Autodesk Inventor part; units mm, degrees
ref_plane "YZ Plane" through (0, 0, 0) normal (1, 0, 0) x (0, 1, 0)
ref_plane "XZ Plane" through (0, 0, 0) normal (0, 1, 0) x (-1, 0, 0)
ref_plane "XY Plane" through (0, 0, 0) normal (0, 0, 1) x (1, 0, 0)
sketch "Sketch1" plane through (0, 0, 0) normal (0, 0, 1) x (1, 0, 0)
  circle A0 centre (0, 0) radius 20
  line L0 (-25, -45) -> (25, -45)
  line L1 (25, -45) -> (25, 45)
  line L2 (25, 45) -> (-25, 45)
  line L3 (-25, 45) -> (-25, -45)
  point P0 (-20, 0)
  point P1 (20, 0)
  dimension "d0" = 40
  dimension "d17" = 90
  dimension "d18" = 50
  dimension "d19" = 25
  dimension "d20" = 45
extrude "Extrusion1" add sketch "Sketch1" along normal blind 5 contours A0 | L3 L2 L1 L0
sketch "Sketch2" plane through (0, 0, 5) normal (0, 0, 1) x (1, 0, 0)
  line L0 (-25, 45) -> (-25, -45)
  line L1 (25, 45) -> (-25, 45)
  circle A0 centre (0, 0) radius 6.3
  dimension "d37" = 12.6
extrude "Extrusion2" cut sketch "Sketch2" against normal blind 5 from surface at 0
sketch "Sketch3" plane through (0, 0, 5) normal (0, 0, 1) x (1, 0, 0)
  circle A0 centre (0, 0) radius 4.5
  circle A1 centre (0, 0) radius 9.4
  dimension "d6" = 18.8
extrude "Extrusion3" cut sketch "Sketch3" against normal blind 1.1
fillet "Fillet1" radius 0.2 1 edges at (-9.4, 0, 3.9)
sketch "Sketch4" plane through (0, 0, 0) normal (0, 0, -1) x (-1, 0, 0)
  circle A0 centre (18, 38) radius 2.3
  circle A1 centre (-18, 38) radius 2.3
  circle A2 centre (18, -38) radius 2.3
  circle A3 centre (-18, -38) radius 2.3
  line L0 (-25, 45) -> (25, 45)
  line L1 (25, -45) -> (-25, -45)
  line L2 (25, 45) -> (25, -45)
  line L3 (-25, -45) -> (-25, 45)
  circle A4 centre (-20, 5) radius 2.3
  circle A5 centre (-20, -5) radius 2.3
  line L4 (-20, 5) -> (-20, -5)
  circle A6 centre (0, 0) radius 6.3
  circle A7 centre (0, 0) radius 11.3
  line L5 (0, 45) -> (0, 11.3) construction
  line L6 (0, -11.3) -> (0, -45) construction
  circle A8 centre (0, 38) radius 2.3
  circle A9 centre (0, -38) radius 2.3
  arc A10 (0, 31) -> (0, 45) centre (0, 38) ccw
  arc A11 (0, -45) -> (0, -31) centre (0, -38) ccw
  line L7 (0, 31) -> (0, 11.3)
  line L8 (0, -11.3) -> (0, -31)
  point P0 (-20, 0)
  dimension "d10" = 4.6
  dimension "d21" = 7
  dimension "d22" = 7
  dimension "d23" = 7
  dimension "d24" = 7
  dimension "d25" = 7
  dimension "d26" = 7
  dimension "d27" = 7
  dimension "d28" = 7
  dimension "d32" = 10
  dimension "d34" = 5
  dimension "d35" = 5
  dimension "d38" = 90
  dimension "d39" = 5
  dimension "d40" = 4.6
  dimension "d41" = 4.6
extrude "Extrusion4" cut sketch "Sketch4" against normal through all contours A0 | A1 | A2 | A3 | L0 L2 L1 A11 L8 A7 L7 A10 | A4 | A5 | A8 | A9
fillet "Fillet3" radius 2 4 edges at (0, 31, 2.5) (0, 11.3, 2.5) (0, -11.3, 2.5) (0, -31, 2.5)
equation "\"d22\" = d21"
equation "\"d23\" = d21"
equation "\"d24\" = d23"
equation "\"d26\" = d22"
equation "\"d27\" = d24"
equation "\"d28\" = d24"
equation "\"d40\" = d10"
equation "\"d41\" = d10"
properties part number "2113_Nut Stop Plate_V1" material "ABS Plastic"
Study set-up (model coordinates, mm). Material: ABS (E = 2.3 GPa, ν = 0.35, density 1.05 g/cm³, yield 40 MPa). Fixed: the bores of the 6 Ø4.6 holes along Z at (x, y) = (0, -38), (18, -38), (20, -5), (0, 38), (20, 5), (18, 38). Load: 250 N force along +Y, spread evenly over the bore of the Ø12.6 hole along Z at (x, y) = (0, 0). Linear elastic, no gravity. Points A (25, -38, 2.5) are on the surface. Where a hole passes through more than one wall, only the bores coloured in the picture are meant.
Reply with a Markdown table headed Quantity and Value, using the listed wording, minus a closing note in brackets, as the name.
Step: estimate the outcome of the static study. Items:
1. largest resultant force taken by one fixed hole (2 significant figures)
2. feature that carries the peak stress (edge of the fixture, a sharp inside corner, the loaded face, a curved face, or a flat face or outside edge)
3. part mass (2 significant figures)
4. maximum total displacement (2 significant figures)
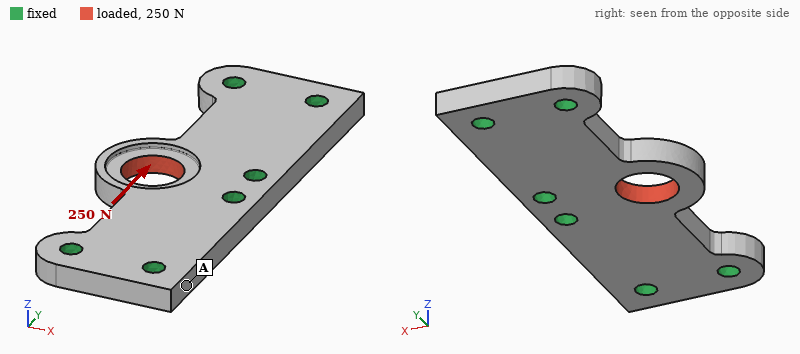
| Quantity | Value |
|---|---|
| largest resultant force taken by one fixed hole | 65 N |
| feature that carries the peak stress | a curved face |
| part mass | 12 g |
| maximum total displacement | 78 µm |
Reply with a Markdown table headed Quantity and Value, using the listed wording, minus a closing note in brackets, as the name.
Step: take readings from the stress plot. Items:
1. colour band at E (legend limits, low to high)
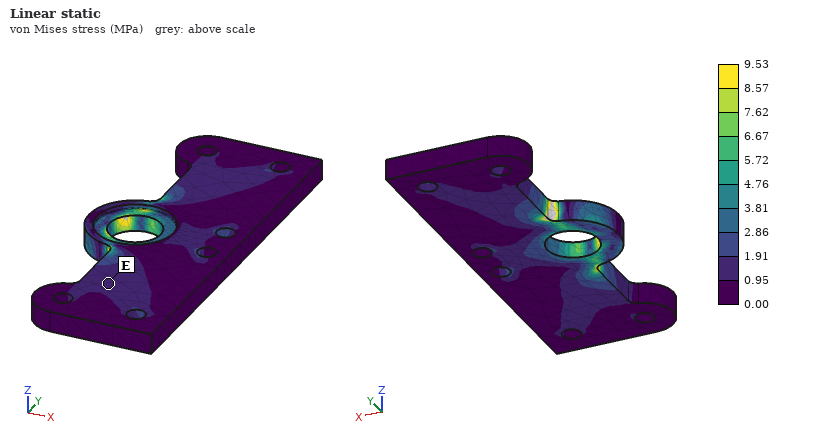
| Quantity | Value |
|---|---|
| colour band at E | 0.95 to 1.91 MPa |
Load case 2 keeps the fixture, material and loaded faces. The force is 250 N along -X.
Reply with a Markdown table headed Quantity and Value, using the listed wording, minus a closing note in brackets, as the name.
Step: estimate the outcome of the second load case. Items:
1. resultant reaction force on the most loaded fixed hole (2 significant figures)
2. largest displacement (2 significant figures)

| Quantity | Value |
|---|---|
| resultant reaction force on the most loaded fixed hole | 100 N |
| largest displacement | 67 µm |
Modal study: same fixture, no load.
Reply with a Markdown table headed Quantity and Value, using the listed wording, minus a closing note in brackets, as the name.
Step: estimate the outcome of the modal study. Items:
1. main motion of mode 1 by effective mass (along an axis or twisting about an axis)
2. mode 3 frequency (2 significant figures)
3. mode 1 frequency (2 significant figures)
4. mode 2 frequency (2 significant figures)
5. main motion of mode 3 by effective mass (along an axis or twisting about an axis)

| Quantity | Value |
|---|---|
| main motion of mode 1 by effective mass | along Z |
| mode 3 frequency | 5500 Hz |
| mode 1 frequency | 2200 Hz |
| mode 2 frequency | 4300 Hz |
| main motion of mode 3 by effective mass | along Z |
